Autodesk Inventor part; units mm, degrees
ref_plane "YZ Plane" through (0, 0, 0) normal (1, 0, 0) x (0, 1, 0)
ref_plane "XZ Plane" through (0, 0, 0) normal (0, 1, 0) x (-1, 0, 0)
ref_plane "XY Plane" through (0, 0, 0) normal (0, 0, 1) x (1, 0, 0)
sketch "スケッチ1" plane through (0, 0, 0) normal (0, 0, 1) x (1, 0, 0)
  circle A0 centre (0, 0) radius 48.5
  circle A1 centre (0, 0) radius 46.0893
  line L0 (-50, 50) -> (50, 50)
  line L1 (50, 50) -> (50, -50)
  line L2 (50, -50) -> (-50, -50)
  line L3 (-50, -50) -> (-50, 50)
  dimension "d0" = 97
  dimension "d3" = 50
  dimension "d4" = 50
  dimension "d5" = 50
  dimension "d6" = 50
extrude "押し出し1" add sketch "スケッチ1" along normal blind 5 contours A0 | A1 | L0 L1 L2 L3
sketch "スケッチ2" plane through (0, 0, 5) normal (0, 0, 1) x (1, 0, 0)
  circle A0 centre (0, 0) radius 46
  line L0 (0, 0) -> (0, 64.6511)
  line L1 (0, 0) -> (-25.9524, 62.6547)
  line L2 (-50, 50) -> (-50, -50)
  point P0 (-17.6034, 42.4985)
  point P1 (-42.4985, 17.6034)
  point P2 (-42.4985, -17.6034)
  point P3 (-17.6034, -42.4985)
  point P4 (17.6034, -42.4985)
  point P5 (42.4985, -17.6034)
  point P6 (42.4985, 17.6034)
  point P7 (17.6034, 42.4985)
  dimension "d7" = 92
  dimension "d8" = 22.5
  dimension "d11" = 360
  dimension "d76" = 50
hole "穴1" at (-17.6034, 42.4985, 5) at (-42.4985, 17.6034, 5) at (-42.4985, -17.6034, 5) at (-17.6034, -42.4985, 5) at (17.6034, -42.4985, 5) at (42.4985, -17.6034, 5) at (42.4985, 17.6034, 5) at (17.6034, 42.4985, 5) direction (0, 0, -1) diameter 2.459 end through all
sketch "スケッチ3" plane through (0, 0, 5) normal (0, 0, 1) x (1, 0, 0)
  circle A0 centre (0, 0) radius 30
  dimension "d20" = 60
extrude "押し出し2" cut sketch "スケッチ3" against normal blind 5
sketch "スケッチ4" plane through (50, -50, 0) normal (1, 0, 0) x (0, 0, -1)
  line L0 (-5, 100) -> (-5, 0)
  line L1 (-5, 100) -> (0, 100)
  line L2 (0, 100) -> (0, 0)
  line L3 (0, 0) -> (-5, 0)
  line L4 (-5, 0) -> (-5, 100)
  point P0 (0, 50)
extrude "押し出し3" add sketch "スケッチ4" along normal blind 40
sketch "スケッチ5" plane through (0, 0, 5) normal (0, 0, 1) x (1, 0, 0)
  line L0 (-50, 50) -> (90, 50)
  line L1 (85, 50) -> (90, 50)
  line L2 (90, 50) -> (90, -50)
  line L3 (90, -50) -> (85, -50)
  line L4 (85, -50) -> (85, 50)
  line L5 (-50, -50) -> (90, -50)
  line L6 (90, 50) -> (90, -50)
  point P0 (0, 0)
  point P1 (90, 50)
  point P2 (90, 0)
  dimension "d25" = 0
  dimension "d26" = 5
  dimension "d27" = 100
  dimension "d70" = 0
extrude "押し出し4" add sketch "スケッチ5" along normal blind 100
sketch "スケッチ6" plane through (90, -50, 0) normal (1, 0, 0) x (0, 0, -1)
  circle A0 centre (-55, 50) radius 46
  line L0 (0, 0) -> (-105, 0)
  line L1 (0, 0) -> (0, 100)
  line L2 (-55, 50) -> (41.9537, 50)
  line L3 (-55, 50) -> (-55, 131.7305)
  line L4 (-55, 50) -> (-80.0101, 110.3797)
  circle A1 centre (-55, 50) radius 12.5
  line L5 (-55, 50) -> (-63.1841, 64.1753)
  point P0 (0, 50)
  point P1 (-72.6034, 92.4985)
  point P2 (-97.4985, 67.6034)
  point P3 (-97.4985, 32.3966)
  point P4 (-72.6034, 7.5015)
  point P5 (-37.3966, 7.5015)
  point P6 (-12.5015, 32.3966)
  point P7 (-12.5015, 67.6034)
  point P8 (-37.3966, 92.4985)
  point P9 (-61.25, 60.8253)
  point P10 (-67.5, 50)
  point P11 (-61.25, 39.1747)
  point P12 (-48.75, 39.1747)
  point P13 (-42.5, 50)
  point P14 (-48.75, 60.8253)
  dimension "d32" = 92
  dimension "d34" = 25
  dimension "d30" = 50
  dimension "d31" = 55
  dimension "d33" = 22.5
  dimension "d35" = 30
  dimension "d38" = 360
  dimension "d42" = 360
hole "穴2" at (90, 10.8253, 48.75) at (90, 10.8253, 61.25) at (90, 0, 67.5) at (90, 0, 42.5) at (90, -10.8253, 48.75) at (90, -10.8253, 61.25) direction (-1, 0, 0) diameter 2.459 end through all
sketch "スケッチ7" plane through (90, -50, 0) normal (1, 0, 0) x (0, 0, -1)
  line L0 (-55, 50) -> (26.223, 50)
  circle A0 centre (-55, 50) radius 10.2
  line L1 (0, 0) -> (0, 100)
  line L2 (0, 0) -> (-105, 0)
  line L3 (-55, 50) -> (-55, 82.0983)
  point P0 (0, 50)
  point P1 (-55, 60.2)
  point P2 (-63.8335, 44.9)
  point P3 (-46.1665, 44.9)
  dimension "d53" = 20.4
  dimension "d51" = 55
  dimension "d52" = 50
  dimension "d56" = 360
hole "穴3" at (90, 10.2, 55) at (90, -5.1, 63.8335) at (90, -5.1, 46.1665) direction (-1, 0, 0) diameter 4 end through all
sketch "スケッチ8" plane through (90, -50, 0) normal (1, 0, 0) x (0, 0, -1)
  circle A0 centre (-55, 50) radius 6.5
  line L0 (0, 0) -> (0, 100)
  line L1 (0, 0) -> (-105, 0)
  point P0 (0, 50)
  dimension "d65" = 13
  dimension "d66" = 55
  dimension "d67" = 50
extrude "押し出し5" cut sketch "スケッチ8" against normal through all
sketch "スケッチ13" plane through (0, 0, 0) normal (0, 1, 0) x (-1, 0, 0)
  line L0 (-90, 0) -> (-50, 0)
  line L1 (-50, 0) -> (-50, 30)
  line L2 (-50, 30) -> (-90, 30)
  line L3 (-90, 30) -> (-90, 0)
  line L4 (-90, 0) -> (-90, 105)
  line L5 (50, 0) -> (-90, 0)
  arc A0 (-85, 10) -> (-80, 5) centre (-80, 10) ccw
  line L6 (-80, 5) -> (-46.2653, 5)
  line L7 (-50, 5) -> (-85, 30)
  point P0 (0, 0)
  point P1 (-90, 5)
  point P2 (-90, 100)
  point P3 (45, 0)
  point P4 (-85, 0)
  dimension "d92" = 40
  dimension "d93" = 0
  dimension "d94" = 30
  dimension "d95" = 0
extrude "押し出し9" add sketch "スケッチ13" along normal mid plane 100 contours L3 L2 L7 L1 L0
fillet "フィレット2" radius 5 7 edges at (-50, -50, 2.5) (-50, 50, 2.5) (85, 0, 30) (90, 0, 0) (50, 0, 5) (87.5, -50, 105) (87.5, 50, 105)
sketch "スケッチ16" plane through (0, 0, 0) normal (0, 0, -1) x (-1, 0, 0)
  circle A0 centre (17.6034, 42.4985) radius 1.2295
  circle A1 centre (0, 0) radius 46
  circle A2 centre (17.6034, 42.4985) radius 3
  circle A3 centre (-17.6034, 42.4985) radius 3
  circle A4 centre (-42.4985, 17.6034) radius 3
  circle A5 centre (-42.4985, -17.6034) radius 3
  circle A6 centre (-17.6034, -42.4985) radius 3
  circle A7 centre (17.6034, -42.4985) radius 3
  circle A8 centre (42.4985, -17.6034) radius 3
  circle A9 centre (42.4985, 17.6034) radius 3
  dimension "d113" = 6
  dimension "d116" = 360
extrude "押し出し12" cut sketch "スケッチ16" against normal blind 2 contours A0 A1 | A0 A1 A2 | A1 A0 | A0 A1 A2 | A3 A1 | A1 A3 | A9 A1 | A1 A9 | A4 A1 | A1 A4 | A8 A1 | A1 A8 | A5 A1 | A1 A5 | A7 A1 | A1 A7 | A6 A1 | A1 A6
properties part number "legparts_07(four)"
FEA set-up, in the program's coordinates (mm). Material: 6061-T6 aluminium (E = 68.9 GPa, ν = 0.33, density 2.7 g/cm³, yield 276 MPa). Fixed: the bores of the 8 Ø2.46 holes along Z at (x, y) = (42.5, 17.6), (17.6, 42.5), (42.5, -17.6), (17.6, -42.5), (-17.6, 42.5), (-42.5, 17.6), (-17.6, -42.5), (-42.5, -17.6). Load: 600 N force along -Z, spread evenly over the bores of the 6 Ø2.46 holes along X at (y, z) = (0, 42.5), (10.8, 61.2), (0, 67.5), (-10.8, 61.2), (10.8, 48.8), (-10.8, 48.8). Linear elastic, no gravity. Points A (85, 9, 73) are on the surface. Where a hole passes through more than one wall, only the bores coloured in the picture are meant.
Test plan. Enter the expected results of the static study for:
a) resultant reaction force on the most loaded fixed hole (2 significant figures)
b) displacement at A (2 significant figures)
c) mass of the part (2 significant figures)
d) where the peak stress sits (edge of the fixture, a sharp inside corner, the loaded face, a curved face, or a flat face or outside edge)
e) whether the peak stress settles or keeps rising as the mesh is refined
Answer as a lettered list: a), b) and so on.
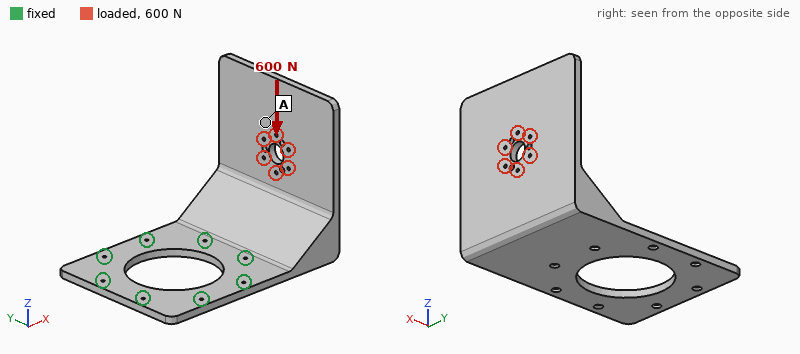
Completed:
a) 780 N
b) 0.58 mm
c) 400 g
d) edge of the fixture
e) keeps rising
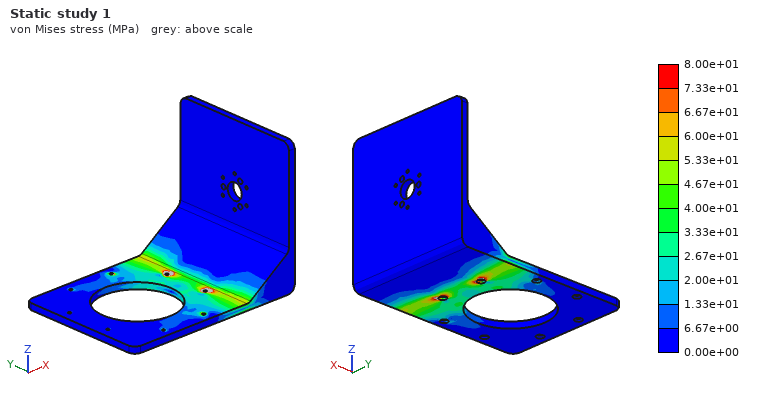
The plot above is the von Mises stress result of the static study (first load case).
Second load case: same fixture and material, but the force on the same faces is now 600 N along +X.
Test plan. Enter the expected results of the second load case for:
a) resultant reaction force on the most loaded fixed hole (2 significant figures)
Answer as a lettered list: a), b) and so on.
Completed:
a) 850 N
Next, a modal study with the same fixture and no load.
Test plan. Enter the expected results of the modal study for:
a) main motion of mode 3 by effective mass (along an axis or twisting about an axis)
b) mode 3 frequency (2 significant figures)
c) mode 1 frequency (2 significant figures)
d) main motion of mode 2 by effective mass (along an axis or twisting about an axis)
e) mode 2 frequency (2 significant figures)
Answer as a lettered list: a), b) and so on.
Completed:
a) along Z
b) 960 Hz
c) 300 Hz
d) along Y
e) 910 Hz
